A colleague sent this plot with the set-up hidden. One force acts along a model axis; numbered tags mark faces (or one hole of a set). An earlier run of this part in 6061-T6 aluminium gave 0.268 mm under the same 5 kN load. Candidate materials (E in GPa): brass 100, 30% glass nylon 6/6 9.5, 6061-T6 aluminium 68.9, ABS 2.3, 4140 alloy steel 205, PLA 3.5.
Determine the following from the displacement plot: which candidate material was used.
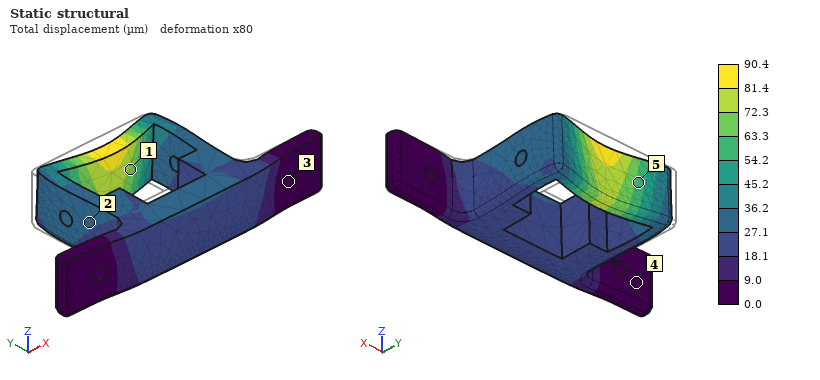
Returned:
4140 alloy steel
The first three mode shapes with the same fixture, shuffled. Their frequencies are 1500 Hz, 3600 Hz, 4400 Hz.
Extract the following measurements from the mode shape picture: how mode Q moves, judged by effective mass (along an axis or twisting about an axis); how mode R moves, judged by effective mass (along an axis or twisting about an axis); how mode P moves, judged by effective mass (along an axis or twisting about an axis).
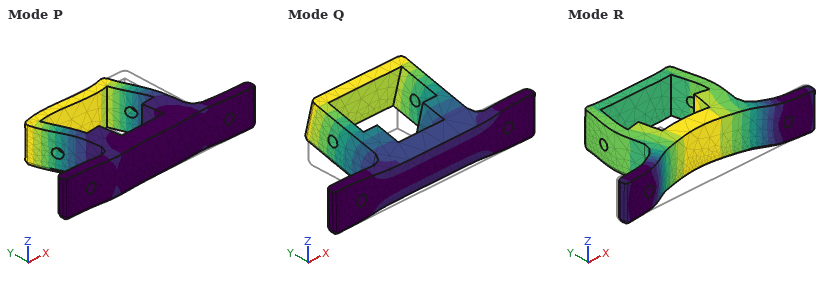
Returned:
along Z
along Y
along X
